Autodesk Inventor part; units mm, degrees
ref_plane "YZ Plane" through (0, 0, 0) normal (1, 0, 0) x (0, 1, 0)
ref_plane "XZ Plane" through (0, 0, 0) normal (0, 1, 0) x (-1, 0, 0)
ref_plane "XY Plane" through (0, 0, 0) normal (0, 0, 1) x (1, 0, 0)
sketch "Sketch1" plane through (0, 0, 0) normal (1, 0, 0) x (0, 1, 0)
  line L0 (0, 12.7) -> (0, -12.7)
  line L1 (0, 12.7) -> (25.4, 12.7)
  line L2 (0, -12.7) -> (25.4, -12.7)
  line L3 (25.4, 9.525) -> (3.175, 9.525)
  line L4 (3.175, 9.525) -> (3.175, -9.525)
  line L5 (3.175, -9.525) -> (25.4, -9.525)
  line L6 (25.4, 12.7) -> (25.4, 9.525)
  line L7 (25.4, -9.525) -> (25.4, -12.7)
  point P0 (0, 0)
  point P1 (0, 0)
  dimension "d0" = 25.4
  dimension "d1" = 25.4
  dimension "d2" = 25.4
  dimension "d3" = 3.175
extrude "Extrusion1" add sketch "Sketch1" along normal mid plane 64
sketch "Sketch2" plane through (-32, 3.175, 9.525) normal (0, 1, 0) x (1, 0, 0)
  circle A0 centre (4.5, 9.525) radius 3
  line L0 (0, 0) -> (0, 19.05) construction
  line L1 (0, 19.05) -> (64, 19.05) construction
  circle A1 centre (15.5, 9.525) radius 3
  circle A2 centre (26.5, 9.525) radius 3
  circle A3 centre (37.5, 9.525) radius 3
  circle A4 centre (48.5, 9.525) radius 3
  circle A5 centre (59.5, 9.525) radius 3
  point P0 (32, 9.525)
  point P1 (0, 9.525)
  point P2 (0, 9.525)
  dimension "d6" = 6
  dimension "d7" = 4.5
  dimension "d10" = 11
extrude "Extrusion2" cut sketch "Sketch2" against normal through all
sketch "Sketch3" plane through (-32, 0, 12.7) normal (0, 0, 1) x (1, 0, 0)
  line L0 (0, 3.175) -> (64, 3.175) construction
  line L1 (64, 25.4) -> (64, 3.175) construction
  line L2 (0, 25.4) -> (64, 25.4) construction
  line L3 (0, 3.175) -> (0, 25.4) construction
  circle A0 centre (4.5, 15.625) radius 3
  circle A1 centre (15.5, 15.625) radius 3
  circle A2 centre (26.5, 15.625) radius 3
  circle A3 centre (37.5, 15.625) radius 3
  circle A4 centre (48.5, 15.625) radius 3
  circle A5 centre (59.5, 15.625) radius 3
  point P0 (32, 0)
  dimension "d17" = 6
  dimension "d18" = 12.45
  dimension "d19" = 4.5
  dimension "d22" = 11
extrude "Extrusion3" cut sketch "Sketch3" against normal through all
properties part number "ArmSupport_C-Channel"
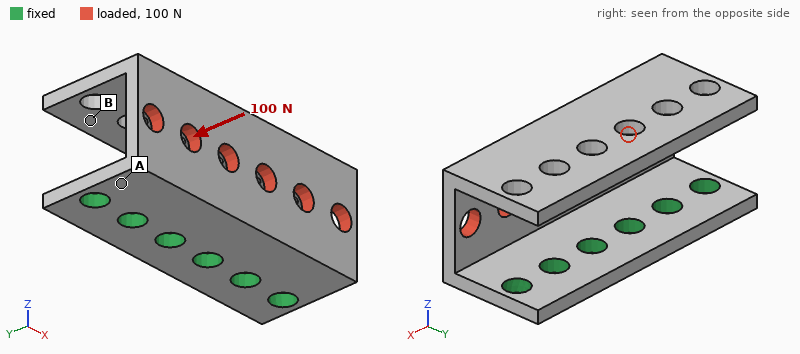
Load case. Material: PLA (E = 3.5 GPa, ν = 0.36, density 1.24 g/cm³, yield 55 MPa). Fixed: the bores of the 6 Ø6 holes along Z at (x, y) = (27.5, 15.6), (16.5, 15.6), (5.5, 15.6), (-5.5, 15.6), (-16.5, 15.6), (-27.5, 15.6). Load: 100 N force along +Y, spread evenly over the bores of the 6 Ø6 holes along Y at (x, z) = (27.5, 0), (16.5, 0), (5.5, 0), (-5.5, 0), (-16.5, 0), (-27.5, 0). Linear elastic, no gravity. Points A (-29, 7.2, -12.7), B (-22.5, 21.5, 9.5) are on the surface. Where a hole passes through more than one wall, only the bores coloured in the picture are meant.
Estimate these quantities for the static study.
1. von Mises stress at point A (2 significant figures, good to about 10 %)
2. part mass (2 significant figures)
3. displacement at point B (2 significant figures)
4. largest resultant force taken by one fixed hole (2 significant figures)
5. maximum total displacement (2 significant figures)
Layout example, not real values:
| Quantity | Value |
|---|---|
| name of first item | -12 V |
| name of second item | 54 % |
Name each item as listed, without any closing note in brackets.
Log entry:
| Quantity | Value |
|---|---|
| von Mises stress at point A | 9.1 MPa |
| part mass | 16 g |
| displacement at point B | 0.70 mm |
| largest resultant force taken by one fixed hole | 18 N |
| maximum total displacement | 0.84 mm |
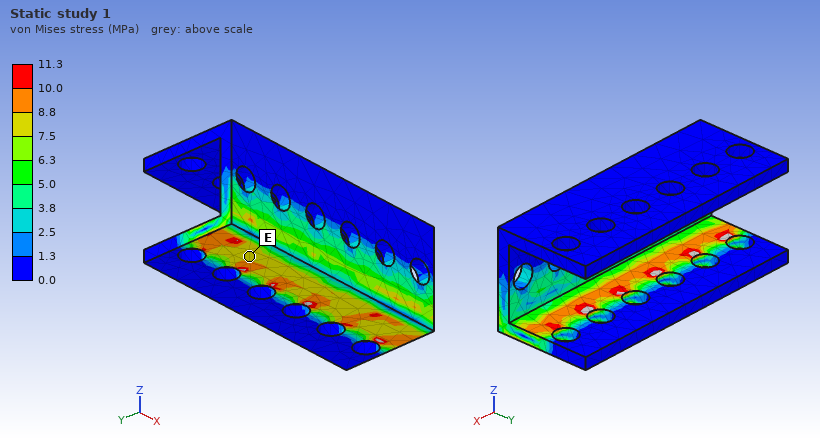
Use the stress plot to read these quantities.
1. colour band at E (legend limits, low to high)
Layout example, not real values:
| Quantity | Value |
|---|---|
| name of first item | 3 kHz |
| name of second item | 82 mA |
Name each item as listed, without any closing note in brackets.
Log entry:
| Quantity | Value |
|---|---|
| colour band at E | 7.5 to 8.8 MPa |
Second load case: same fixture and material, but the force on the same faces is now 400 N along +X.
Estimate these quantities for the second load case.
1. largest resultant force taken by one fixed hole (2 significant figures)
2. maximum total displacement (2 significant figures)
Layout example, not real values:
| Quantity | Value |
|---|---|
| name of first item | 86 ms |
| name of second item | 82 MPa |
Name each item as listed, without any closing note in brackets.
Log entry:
| Quantity | Value |
|---|---|
| largest resultant force taken by one fixed hole | 110 N |
| maximum total displacement | 0.53 mm |
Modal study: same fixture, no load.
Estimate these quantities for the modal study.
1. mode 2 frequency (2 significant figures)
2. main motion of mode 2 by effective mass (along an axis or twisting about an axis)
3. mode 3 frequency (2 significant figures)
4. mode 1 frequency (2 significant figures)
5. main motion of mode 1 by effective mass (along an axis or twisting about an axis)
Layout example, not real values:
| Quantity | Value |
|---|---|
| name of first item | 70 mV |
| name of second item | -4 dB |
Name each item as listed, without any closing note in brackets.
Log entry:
| Quantity | Value |
|---|---|
| mode 2 frequency | 700 Hz |
| main motion of mode 2 by effective mass | along X |
| mode 3 frequency | 1100 Hz |
| mode 1 frequency | 420 Hz |
| main motion of mode 1 by effective mass | along Y |
